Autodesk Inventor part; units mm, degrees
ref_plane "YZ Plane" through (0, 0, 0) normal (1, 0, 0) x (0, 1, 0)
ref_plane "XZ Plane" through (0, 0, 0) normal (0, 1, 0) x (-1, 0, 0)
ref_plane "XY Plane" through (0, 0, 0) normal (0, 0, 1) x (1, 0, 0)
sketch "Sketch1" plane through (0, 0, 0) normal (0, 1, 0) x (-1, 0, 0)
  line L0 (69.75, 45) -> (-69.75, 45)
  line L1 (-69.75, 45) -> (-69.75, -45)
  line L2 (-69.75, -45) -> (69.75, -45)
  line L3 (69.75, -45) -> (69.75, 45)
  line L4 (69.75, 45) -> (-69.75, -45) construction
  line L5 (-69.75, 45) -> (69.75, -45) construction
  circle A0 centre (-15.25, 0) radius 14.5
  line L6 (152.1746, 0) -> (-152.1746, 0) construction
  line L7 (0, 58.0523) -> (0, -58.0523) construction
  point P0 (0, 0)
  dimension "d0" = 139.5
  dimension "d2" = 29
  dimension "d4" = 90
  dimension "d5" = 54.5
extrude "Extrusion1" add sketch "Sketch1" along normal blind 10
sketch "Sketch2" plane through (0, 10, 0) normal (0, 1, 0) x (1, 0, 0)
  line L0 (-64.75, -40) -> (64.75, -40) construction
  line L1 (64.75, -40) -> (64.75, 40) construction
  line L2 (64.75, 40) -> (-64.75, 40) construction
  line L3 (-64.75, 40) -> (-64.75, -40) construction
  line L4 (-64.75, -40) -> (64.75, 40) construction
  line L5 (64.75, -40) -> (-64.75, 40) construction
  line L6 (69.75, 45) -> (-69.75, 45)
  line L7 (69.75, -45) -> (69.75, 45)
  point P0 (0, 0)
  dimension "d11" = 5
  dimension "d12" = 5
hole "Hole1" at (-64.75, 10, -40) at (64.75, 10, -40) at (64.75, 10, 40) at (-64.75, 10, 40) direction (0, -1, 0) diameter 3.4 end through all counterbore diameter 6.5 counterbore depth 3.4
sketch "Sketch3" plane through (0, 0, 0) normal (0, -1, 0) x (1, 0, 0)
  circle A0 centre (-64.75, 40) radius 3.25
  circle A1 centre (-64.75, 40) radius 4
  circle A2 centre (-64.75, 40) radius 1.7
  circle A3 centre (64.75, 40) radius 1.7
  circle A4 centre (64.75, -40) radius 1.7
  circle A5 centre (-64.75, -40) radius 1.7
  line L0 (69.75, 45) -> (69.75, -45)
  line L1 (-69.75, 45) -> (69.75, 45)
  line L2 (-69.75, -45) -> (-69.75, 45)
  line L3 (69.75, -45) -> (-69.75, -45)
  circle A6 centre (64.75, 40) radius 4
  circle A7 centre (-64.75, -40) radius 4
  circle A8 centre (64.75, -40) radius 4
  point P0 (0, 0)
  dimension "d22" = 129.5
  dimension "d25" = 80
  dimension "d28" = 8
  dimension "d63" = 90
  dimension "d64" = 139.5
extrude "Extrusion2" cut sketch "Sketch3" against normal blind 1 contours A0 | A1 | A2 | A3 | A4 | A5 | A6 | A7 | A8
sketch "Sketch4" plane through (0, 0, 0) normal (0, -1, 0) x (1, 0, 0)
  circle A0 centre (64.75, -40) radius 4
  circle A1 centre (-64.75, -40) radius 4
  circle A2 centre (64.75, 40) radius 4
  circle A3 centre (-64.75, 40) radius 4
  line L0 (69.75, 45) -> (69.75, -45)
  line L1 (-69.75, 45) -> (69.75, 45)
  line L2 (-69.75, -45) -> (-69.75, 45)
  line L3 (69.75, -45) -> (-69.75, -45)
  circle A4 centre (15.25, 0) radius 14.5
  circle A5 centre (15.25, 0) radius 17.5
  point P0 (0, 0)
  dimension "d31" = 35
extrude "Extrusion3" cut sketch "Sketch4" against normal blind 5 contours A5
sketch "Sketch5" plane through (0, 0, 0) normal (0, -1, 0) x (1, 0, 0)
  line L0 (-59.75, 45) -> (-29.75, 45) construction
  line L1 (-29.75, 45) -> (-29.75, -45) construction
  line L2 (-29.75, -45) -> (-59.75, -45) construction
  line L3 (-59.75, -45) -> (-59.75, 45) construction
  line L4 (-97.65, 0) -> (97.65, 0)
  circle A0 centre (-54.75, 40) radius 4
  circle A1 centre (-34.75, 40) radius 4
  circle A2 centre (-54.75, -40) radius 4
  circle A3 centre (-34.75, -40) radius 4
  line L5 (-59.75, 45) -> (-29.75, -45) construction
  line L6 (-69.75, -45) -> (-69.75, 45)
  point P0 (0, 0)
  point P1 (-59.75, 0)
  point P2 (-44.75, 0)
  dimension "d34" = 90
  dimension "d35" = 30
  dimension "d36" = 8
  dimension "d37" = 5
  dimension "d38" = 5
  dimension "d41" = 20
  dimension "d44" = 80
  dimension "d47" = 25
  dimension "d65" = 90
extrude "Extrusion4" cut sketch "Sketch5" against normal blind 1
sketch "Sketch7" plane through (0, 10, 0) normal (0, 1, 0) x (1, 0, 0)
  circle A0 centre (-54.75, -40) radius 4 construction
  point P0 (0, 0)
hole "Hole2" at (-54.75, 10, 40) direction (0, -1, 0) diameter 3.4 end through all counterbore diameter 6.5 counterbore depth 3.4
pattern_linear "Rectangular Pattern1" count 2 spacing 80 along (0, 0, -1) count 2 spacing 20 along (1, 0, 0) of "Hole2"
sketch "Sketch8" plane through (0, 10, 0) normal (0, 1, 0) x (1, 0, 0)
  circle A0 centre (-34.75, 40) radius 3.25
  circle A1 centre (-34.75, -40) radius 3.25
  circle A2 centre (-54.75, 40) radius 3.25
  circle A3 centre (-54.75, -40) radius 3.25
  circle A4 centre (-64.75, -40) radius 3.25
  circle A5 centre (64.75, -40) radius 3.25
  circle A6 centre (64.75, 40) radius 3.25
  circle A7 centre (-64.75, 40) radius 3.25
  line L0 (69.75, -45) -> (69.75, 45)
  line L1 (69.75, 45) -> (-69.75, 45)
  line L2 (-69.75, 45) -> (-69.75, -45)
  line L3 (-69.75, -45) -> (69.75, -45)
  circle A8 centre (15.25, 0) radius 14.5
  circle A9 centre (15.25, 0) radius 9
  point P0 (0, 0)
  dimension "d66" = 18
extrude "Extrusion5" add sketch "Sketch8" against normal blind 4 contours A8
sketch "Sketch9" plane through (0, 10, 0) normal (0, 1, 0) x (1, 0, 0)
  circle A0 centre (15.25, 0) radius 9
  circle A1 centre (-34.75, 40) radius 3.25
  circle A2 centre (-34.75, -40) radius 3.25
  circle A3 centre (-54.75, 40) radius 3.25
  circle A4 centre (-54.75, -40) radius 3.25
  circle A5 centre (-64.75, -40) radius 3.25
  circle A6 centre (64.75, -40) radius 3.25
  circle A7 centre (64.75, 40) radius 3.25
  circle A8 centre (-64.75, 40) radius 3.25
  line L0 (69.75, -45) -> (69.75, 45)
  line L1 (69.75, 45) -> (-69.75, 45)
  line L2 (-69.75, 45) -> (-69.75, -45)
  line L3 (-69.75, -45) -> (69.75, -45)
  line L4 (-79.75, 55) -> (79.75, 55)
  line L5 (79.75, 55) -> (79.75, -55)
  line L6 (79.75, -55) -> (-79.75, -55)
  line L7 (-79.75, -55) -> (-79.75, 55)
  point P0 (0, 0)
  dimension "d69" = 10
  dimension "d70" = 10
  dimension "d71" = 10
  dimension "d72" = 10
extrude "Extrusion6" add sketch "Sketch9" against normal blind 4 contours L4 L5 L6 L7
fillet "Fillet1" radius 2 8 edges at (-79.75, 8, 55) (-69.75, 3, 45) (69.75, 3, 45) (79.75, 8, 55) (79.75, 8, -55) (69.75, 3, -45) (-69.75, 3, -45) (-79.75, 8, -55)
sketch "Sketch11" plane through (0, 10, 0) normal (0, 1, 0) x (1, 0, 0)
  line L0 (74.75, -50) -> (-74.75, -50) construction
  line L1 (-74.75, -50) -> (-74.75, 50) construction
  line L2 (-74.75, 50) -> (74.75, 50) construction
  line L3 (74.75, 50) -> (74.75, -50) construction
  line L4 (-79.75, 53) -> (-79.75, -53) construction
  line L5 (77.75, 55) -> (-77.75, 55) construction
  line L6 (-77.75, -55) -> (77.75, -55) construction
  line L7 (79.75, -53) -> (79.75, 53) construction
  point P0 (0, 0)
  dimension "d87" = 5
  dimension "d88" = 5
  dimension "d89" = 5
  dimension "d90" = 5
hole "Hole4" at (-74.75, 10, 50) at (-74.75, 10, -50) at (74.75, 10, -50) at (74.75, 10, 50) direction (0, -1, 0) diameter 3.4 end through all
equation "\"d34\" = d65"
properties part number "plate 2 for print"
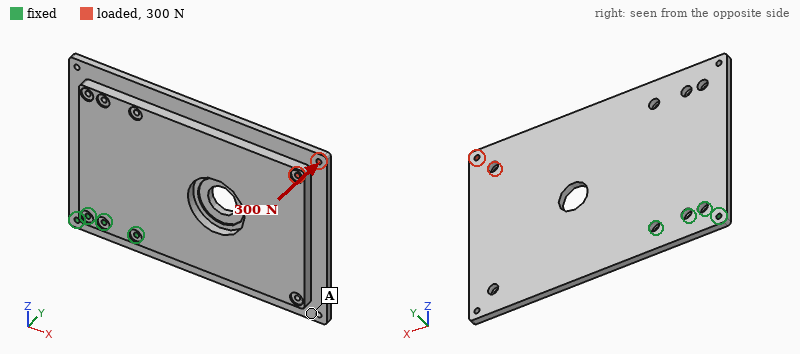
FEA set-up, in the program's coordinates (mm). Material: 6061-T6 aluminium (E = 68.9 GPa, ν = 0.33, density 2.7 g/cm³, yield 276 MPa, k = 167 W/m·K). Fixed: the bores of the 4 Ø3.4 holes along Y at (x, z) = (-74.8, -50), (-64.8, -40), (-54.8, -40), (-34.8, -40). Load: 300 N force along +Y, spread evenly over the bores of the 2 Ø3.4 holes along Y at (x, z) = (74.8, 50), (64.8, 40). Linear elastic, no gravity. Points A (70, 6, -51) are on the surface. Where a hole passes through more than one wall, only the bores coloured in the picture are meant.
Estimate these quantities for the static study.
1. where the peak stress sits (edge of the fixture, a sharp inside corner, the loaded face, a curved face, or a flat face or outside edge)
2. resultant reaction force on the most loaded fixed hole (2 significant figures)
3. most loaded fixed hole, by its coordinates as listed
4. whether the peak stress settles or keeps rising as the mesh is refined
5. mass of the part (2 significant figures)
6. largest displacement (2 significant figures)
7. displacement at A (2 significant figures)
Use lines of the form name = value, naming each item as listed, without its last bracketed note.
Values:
where the peak stress sits = edge of the fixture
resultant reaction force on the most loaded fixed hole = 1.2 kN
most loaded fixed hole, by its coordinates as listed = (-34.8, -40)
whether the peak stress settles or keeps rising as the mesh is refined = keeps rising
mass of the part = 370 g
largest displacement = 1.0 mm
displacement at A = 0.32 mm
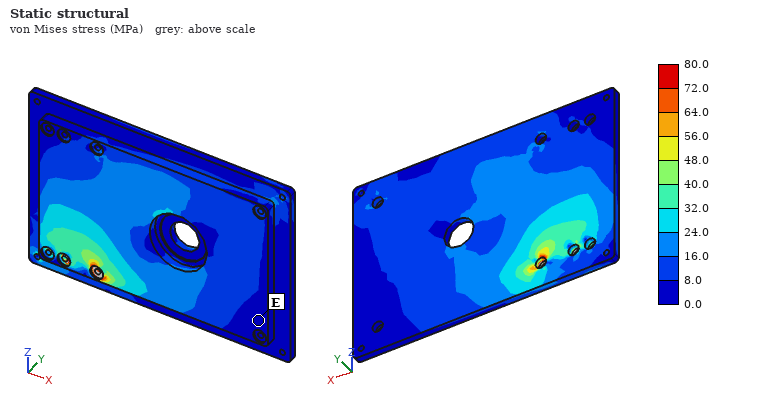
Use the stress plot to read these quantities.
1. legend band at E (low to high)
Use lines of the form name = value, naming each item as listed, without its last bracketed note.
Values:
legend band at E = 0.0 to 8.0 MPa
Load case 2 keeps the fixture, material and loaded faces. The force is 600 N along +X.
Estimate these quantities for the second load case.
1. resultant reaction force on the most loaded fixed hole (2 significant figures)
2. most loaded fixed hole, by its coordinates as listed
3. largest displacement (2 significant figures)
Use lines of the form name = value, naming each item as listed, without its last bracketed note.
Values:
resultant reaction force on the most loaded fixed hole = 1.5 kN
most loaded fixed hole, by its coordinates as listed = (-34.8, -40)
largest displacement = 50 µm
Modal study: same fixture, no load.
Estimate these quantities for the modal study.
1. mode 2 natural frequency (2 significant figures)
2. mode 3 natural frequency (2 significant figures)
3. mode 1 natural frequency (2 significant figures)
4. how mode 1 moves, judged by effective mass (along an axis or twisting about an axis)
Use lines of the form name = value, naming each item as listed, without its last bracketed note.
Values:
mode 2 natural frequency = 700 Hz
mode 3 natural frequency = 1400 Hz
mode 1 natural frequency = 360 Hz
how mode 1 moves, judged by effective mass = along Y
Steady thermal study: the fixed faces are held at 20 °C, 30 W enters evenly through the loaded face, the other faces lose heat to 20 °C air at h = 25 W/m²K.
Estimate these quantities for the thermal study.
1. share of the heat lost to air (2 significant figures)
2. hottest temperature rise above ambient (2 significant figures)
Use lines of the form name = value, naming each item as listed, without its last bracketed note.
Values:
share of the heat lost to air = 40 %
hottest temperature rise above ambient = 48 K
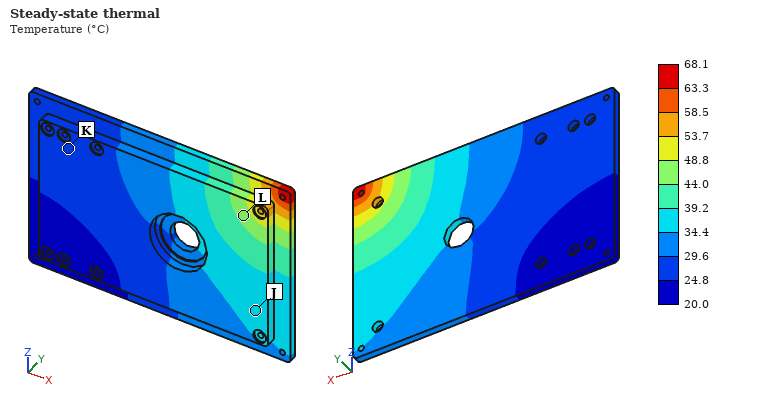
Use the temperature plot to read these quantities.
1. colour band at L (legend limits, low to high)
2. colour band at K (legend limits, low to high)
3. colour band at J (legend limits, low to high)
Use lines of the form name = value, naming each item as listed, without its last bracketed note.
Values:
colour band at L = 44.0 to 48.8 °C
colour band at K = 24.8 to 29.6 °C
colour band at J = 34.4 to 39.2 °C
